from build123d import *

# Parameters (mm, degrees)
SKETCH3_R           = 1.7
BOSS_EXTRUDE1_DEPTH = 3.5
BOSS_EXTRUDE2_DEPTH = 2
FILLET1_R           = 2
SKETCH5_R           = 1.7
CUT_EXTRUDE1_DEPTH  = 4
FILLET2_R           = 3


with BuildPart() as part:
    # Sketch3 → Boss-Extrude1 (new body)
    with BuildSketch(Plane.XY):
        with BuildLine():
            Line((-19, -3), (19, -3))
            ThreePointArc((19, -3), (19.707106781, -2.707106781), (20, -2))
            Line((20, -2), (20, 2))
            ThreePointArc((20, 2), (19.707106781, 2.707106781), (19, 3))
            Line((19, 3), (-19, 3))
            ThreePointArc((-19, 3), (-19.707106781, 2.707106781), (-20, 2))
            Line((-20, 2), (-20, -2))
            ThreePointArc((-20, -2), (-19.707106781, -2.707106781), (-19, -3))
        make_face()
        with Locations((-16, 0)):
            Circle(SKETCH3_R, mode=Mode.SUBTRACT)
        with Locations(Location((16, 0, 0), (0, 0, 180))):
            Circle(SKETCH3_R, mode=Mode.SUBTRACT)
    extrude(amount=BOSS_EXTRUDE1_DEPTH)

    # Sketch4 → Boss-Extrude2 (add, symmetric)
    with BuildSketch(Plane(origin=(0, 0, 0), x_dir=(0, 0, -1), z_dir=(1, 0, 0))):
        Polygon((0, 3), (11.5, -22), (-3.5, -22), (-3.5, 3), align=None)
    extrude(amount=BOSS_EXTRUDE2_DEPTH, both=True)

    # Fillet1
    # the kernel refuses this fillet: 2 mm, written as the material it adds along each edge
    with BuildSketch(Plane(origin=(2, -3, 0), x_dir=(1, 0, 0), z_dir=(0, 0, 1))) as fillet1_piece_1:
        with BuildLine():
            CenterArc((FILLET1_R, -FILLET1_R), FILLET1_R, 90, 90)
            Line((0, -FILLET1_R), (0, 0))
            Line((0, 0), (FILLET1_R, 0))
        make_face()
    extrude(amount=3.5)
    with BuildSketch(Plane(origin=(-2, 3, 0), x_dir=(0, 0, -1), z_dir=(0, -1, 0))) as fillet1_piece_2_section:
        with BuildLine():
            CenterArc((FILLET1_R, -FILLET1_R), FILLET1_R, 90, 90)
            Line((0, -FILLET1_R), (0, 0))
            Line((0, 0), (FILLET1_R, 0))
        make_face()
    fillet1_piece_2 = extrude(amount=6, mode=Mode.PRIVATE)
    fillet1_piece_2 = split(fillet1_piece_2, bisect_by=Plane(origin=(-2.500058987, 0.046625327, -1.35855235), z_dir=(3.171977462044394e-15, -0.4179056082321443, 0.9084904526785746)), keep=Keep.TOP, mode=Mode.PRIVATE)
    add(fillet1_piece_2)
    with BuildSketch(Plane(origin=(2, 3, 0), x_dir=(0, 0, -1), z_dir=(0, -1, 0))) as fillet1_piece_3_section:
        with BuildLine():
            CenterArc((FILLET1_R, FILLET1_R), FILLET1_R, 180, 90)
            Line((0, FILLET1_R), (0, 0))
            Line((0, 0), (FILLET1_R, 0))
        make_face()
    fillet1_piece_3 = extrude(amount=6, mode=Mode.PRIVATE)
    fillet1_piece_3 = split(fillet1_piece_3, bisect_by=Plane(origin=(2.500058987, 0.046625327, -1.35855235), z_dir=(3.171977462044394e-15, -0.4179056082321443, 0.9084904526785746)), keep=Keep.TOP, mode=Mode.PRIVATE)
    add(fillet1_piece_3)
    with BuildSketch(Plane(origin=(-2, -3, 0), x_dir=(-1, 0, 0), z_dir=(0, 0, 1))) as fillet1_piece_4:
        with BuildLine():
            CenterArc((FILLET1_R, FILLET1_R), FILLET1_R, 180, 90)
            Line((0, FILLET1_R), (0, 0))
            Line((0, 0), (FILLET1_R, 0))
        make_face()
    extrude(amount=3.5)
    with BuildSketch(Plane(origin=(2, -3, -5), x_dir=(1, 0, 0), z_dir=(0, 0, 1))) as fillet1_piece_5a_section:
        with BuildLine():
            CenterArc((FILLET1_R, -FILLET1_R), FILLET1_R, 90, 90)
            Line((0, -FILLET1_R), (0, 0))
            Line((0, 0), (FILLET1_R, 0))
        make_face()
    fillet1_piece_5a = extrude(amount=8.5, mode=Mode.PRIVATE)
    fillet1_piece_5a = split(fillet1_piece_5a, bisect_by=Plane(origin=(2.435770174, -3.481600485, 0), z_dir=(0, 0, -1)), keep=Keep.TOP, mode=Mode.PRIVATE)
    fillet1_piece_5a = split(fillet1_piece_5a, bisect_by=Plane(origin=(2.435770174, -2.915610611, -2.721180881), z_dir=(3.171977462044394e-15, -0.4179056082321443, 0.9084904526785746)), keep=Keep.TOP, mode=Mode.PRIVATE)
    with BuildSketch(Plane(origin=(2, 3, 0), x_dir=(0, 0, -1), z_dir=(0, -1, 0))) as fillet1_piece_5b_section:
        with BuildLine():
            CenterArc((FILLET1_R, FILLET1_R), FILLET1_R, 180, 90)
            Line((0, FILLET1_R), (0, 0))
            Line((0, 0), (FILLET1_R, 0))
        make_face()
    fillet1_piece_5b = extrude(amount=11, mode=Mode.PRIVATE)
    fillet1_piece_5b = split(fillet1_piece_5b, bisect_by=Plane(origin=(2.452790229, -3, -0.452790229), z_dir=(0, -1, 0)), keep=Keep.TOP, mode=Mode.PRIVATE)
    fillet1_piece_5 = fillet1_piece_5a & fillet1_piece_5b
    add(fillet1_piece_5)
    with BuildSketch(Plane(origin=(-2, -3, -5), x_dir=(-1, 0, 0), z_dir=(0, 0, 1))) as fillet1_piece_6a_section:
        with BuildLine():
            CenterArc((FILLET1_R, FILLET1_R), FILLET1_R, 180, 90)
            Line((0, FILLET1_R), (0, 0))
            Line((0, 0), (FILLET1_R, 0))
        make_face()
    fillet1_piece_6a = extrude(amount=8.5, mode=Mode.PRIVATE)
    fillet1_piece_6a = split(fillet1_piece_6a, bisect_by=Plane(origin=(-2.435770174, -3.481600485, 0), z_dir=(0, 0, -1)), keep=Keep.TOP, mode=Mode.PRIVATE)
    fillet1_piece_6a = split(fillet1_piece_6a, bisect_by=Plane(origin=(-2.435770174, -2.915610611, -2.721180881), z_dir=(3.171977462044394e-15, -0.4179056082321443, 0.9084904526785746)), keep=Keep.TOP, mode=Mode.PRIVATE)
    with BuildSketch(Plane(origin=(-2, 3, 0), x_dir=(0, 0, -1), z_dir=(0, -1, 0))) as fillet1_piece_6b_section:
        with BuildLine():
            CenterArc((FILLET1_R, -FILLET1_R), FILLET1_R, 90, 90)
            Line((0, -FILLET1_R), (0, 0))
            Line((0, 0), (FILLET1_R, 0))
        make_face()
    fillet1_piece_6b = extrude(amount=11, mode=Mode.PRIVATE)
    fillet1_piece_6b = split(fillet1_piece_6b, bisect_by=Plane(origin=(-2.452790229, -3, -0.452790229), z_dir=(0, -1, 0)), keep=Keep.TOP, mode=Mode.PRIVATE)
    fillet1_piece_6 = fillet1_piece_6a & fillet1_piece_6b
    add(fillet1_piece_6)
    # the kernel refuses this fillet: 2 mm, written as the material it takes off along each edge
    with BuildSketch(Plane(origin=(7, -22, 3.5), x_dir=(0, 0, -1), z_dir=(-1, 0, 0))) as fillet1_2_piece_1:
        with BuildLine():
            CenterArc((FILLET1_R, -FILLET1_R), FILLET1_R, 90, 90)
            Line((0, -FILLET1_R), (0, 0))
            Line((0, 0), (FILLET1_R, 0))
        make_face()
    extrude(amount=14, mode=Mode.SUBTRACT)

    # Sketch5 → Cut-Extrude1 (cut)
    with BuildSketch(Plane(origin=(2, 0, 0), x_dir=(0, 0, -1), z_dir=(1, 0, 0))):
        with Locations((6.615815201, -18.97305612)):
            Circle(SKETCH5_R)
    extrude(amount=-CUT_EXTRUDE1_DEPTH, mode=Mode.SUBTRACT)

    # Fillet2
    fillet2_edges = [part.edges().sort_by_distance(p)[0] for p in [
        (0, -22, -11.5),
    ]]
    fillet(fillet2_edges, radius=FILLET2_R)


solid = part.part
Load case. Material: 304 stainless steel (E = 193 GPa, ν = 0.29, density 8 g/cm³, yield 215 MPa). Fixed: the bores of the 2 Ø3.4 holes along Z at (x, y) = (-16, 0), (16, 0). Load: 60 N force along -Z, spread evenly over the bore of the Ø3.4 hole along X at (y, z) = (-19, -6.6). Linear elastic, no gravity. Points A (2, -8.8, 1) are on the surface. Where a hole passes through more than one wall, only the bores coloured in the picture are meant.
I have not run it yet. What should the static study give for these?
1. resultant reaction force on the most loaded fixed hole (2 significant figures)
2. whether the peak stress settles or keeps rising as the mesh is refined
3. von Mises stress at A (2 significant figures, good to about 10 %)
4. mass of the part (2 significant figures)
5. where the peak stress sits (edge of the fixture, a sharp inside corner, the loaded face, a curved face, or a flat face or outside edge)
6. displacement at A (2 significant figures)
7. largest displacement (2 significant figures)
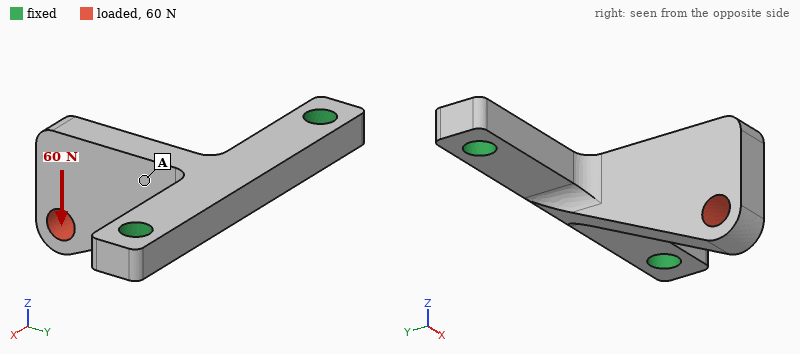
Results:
33 N
keeps rising
8.7 MPa
13 g
edge of the fixture
19 µm
52 µm
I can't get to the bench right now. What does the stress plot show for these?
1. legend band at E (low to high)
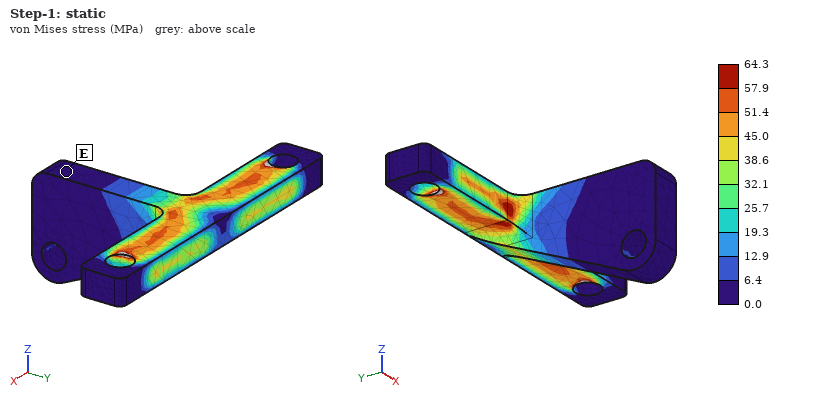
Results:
0.0 to 6.4 MPa
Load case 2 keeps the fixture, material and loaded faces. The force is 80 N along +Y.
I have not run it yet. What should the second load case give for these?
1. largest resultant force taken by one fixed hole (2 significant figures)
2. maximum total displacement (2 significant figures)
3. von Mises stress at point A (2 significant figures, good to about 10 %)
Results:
40 N
31 µm
3.5 MPa
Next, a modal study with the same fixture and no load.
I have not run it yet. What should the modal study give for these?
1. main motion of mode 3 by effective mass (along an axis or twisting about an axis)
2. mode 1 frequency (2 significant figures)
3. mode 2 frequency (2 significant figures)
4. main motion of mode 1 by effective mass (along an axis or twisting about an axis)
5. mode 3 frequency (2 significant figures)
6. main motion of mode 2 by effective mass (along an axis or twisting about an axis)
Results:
along Y
3100 Hz
5600 Hz
along Z
13 kHz
along X
